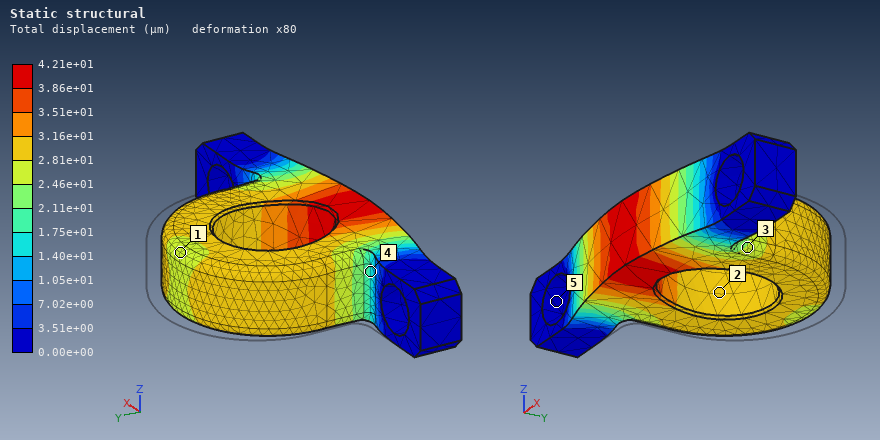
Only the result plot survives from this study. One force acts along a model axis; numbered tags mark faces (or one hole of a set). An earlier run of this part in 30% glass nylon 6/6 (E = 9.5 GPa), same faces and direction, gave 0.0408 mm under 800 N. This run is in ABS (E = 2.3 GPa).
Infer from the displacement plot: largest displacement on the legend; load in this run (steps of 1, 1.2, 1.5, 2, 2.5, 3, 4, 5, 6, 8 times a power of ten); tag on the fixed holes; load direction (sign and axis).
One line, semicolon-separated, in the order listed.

4.21e+01 µm; 200 N; 5; -Y
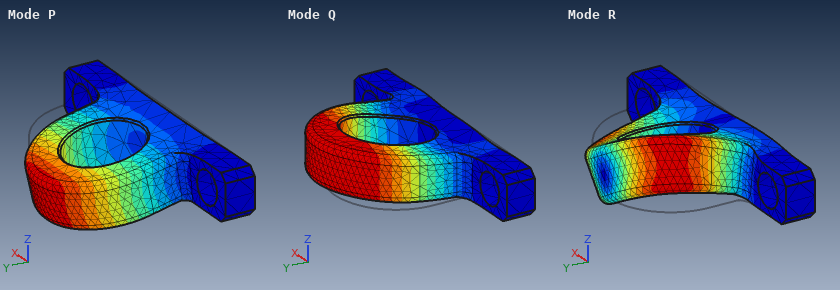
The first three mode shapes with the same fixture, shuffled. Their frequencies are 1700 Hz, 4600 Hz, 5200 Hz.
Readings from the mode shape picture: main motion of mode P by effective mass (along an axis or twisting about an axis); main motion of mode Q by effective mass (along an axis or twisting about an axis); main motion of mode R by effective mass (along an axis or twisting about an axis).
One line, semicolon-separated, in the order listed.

along Z; along X; twisting about Y
